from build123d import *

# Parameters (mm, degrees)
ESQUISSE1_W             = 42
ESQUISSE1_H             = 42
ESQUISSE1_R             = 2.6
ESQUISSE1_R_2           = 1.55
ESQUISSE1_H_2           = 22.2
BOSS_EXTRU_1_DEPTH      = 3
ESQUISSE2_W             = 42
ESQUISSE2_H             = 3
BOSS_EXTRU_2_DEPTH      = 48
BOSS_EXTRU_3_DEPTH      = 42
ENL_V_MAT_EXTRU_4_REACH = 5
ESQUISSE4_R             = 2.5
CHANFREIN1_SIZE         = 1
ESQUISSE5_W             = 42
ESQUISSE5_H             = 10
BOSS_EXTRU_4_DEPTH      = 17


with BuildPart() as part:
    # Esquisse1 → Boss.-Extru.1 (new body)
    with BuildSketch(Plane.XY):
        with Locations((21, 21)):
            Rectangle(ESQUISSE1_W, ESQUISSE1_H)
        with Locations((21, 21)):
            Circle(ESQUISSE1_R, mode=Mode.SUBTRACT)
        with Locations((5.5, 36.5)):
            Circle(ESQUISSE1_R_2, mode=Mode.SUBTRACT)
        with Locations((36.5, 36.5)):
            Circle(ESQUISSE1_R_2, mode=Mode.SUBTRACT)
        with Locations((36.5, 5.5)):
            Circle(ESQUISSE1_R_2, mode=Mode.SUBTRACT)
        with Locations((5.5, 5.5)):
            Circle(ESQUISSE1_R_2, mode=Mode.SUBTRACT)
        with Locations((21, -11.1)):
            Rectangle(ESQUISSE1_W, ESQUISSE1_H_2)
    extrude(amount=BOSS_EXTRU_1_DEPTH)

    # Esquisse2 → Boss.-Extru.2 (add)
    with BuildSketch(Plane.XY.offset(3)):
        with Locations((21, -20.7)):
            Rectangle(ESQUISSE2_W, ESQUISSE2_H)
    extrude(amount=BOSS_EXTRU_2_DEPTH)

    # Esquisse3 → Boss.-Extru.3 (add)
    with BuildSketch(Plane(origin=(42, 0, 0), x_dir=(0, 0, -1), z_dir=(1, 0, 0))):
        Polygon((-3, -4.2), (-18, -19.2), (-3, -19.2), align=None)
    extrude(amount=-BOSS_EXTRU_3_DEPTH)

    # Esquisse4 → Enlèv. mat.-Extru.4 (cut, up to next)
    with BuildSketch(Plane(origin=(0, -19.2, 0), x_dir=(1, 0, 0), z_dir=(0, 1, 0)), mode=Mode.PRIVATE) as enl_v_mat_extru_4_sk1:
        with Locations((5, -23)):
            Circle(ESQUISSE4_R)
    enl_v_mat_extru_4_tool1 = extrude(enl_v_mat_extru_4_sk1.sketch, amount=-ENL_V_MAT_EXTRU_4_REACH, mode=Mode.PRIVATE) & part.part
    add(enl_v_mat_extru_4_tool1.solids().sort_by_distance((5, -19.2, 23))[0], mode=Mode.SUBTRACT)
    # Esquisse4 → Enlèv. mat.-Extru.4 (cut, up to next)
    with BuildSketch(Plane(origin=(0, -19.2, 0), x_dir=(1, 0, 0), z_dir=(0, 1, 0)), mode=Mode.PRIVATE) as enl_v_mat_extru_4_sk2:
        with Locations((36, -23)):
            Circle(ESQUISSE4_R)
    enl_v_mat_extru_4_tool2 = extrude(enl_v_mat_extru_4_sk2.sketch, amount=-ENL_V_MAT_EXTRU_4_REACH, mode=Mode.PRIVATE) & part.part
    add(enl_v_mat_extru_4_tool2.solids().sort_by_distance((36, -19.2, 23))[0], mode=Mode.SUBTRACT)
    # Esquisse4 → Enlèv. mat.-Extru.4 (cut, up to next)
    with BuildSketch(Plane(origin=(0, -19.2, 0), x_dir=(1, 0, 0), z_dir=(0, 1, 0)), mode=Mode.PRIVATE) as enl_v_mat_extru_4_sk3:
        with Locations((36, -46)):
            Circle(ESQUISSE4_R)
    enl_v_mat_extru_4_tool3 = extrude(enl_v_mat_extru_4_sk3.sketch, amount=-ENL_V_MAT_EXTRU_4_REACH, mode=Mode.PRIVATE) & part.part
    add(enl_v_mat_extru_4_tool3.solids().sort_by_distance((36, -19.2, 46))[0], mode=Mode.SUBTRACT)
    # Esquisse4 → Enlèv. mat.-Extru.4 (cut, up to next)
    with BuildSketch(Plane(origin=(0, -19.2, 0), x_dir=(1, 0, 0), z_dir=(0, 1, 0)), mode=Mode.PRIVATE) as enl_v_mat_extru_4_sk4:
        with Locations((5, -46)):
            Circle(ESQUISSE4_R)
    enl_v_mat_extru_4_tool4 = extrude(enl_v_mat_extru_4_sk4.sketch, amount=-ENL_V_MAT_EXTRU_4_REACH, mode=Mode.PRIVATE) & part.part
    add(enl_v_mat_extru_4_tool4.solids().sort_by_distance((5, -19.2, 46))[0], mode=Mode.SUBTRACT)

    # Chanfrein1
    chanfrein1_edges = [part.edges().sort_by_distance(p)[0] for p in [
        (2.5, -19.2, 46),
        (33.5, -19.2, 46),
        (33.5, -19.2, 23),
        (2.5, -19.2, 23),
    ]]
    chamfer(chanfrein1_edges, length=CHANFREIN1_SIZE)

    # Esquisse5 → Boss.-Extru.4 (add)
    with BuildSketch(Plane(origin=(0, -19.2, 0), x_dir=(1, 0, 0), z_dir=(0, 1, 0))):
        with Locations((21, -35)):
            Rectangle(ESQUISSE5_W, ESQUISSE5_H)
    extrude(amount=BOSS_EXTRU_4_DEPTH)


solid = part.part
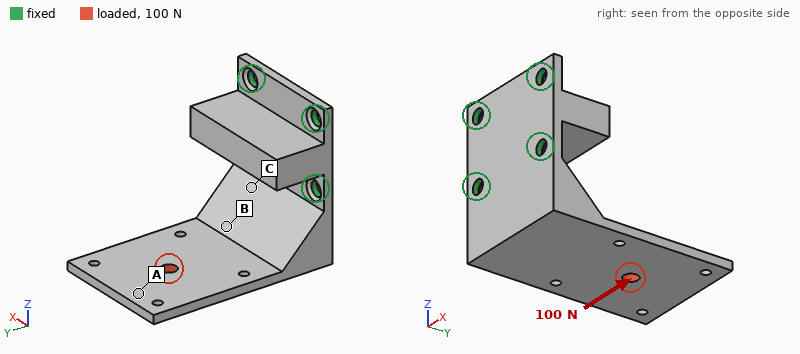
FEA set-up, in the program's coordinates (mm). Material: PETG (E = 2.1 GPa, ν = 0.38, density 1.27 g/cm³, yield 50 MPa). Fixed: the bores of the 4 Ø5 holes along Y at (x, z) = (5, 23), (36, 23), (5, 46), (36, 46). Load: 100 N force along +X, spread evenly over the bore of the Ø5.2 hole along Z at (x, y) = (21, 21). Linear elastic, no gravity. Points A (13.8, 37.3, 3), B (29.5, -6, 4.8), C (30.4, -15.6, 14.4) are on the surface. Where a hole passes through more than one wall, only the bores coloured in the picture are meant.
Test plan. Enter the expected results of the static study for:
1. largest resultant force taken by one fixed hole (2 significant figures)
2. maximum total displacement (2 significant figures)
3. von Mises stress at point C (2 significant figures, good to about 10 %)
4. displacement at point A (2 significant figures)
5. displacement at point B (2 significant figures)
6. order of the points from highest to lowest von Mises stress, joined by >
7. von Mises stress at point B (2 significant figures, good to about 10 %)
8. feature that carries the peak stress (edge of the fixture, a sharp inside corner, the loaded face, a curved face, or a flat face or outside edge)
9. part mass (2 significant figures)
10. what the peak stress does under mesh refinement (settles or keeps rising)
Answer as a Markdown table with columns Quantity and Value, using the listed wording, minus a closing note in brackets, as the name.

| Quantity | Value |
|---|---|
| largest resultant force taken by one fixed hole | 160 N |
| maximum total displacement | 0.94 mm |
| von Mises stress at point C | 7.1 MPa |
| displacement at point A | 0.81 mm |
| displacement at point B | 0.20 mm |
| order of the points from highest to lowest von Mises stress, joined by > | C > B > A |
| von Mises stress at point B | 4.0 MPa |
| feature that carries the peak stress | edge of the fixture |
| part mass | 32 g |
| what the peak stress does under mesh refinement | keeps rising |
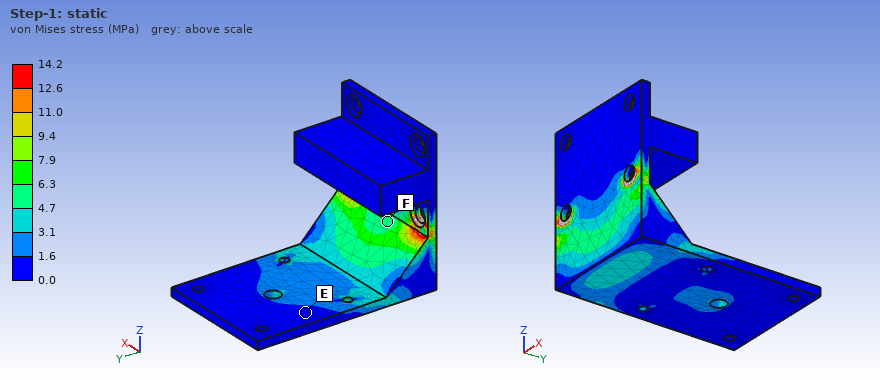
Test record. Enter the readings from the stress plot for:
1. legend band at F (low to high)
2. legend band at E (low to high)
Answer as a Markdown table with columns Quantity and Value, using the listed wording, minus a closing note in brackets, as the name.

| Quantity | Value |
|---|---|
| legend band at F | 4.7 to 6.3 MPa |
| legend band at E | 0.0 to 1.6 MPa |
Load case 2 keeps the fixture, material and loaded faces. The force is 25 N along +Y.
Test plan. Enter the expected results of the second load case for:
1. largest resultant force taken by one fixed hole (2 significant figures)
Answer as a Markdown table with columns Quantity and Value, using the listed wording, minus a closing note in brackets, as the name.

| Quantity | Value |
|---|---|
| largest resultant force taken by one fixed hole | 18 N |
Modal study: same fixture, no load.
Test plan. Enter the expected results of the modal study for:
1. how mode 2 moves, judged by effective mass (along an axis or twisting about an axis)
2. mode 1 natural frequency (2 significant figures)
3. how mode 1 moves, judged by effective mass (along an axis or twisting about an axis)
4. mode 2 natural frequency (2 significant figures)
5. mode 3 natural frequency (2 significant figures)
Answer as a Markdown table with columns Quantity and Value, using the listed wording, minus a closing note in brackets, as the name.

| Quantity | Value |
|---|---|
| how mode 2 moves, judged by effective mass | along Y |
| mode 1 natural frequency | 170 Hz |
| how mode 1 moves, judged by effective mass | along Z |
| mode 2 natural frequency | 540 Hz |
| mode 3 natural frequency | 650 Hz |
